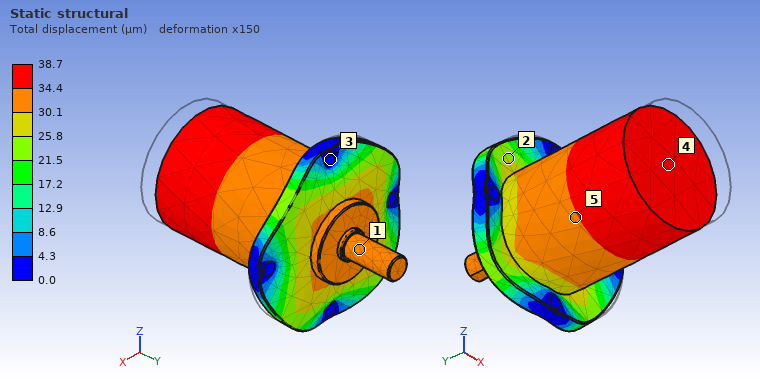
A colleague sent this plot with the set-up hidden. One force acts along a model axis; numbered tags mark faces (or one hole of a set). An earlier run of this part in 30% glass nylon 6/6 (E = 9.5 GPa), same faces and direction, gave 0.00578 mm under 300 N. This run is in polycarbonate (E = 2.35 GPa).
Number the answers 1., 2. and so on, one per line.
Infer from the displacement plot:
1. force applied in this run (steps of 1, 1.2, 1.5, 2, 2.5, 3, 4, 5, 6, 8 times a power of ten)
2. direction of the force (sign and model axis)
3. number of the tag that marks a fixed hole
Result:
1. 500 N
2. +Y
3. 3
